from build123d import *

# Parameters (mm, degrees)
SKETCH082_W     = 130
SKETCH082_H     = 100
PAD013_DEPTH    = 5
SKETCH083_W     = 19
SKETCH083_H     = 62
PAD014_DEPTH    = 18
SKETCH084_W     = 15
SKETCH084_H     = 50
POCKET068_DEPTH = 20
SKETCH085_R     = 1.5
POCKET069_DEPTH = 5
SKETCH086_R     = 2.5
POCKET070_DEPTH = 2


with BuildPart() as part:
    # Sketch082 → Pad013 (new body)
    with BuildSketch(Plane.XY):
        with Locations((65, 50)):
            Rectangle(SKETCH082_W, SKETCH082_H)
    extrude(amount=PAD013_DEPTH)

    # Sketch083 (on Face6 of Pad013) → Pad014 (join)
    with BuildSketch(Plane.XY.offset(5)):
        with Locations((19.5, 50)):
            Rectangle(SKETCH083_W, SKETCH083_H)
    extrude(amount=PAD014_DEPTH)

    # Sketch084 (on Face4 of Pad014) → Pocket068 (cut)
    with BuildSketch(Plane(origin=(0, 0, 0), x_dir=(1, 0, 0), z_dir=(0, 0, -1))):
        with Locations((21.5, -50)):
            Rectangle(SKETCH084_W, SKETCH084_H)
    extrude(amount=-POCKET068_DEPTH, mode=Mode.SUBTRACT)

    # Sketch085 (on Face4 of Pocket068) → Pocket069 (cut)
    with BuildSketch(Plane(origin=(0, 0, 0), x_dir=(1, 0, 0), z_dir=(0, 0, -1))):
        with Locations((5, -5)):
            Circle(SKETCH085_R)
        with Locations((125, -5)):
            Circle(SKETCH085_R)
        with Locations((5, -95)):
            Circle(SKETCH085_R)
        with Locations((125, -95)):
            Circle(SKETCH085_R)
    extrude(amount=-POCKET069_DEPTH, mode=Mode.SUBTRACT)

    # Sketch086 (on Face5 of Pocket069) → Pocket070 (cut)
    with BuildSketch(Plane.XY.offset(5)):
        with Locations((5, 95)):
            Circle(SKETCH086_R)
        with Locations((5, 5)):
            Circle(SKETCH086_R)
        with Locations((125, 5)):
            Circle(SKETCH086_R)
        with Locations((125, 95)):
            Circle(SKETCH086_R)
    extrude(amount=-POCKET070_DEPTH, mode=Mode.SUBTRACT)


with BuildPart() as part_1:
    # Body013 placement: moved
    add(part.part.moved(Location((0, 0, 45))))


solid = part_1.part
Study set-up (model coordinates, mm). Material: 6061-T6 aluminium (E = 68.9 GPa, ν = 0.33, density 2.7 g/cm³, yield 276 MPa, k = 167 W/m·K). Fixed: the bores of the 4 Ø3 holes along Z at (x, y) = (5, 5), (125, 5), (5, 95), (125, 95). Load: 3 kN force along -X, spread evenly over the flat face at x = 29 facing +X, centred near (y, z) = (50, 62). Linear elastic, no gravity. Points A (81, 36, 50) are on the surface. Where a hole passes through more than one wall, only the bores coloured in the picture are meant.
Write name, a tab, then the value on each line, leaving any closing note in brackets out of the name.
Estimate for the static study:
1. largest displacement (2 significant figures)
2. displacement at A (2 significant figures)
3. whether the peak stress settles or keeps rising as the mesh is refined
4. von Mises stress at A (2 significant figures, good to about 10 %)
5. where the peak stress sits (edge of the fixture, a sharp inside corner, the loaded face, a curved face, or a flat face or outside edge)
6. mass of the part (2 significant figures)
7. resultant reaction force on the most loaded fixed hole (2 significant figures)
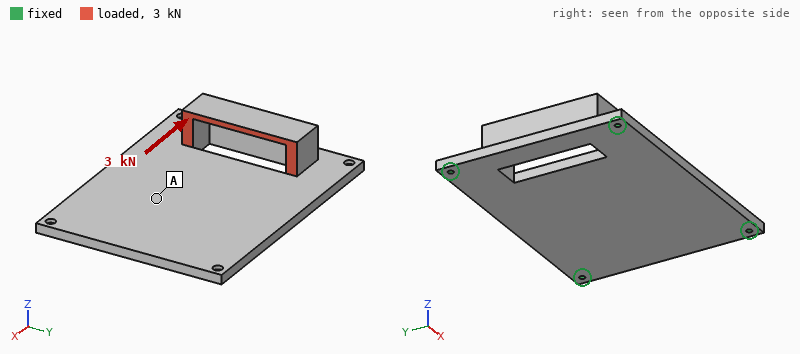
largest displacement	0.34 mm
displacement at A	0.20 mm
whether the peak stress settles or keeps rising as the mesh is refined	keeps rising
von Mises stress at A	14 MPa
where the peak stress sits	edge of the fixture
mass of the part	190 g
resultant reaction force on the most loaded fixed hole	1.0 kN
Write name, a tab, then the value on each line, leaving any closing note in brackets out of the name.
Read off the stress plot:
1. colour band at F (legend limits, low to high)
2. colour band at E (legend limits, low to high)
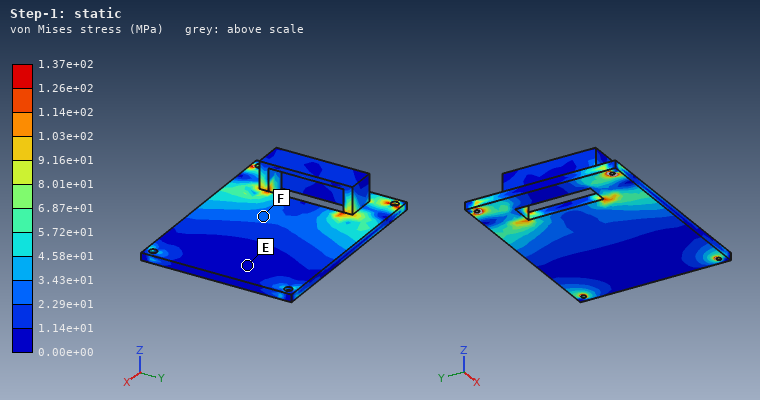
colour band at F	2.29e+01 to 3.43e+01 MPa
colour band at E	0.00e+00 to 1.14e+01 MPa
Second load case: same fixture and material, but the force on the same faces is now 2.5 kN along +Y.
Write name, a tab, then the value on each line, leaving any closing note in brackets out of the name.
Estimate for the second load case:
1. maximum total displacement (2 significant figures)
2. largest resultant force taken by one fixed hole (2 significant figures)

maximum total displacement	62 µm
largest resultant force taken by one fixed hole	1.2 kN
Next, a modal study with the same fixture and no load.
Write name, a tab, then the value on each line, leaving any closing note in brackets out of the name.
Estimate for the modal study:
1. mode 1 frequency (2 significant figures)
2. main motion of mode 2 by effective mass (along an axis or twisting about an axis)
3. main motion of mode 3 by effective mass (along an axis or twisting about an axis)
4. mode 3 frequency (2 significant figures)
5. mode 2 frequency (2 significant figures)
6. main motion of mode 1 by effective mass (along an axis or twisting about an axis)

mode 1 frequency	1100 Hz
main motion of mode 2 by effective mass	twisting about X
main motion of mode 3 by effective mass	twisting about Y
mode 3 frequency	2500 Hz
mode 2 frequency	2000 Hz
main motion of mode 1 by effective mass	along Z
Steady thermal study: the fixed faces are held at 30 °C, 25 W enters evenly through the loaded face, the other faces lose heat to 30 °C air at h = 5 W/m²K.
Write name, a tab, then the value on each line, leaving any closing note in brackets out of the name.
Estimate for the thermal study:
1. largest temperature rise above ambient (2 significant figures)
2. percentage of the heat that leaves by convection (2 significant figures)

largest temperature rise above ambient	23 K
percentage of the heat that leaves by convection	5.0 %
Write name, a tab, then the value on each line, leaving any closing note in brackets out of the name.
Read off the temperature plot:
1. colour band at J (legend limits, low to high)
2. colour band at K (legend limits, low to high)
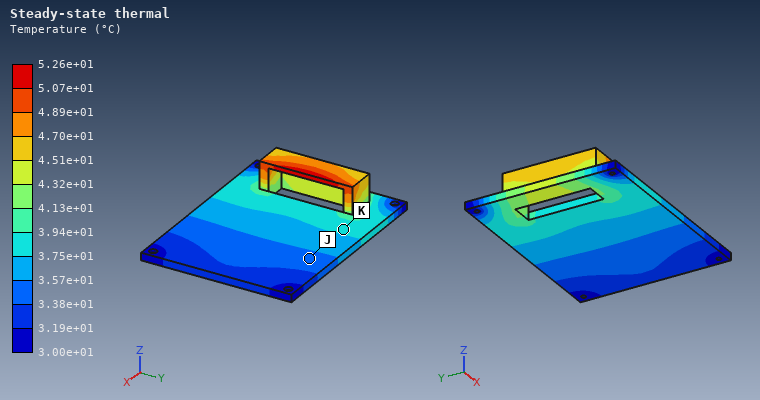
colour band at J	3.38e+01 to 3.57e+01 °C
colour band at K	3.75e+01 to 3.94e+01 °C
